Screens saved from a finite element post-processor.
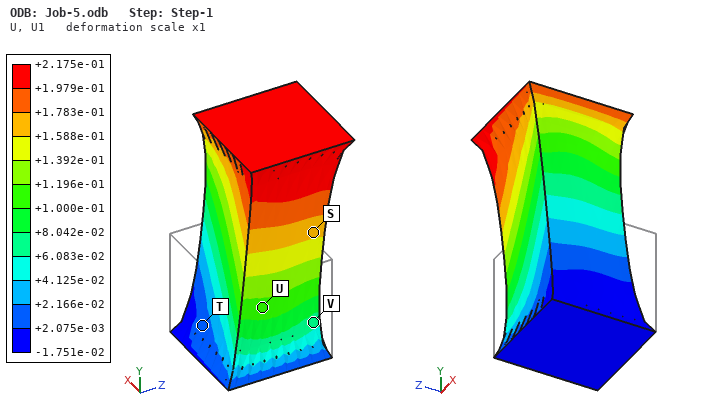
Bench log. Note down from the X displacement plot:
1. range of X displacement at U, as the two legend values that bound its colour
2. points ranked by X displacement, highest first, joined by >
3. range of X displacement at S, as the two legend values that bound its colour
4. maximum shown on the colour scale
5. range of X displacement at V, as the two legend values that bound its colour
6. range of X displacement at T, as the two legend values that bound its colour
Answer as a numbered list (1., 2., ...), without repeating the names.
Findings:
1. +1.000e-01 to +1.196e-01
2. S > U > V > T
3. +1.588e-01 to +1.783e-01
4. +2.175e-01
5. +6.083e-02 to +8.042e-02
6. +2.075e-03 to +2.166e-02
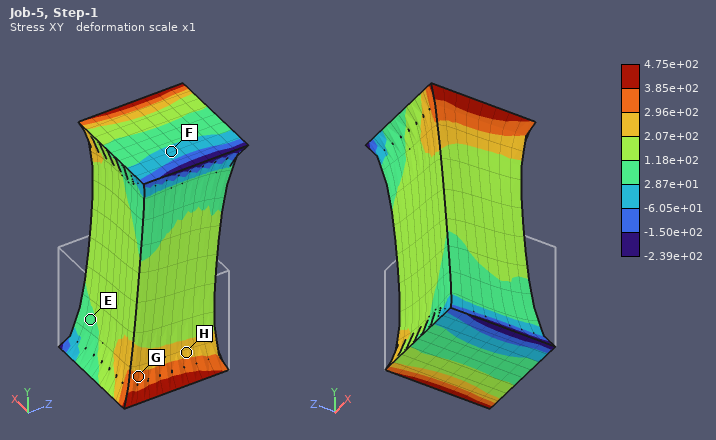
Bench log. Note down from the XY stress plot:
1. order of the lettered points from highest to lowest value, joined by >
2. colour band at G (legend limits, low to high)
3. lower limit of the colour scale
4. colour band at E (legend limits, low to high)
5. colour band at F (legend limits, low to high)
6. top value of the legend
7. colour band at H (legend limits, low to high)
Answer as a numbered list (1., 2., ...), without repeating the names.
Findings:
1. G > H > E > F
2. 2.96e+02 to 3.85e+02
3. -2.39e+02
4. 2.87e+01 to 1.18e+02
5. -6.05e+01 to 2.87e+01
6. 4.75e+02
7. 2.07e+02 to 2.96e+02
